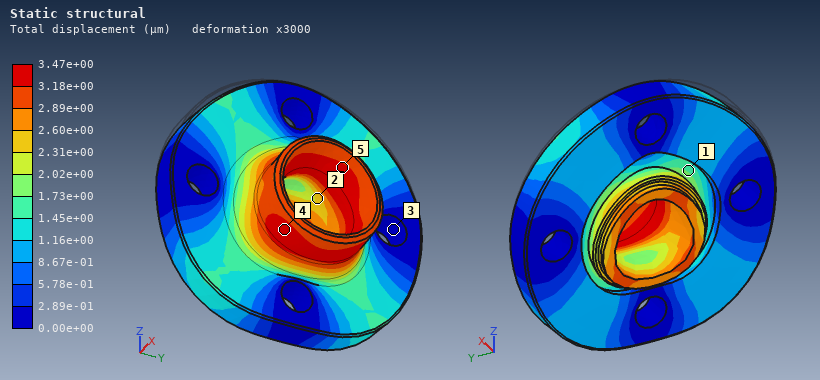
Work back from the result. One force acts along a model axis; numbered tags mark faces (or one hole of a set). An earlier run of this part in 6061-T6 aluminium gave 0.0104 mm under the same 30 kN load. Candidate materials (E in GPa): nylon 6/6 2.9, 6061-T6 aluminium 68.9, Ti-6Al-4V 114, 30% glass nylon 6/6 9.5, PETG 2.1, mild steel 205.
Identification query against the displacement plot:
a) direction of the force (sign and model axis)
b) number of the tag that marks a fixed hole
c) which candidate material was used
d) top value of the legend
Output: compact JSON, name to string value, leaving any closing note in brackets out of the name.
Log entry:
{"direction of the force": "-Z", "number of the tag that marks a fixed hole": "3", "which candidate material was used": "mild steel", "top value of the legend": "3.47e+00 µm"}
